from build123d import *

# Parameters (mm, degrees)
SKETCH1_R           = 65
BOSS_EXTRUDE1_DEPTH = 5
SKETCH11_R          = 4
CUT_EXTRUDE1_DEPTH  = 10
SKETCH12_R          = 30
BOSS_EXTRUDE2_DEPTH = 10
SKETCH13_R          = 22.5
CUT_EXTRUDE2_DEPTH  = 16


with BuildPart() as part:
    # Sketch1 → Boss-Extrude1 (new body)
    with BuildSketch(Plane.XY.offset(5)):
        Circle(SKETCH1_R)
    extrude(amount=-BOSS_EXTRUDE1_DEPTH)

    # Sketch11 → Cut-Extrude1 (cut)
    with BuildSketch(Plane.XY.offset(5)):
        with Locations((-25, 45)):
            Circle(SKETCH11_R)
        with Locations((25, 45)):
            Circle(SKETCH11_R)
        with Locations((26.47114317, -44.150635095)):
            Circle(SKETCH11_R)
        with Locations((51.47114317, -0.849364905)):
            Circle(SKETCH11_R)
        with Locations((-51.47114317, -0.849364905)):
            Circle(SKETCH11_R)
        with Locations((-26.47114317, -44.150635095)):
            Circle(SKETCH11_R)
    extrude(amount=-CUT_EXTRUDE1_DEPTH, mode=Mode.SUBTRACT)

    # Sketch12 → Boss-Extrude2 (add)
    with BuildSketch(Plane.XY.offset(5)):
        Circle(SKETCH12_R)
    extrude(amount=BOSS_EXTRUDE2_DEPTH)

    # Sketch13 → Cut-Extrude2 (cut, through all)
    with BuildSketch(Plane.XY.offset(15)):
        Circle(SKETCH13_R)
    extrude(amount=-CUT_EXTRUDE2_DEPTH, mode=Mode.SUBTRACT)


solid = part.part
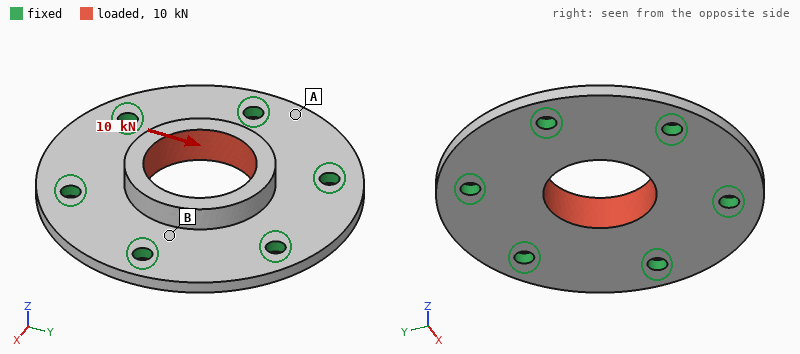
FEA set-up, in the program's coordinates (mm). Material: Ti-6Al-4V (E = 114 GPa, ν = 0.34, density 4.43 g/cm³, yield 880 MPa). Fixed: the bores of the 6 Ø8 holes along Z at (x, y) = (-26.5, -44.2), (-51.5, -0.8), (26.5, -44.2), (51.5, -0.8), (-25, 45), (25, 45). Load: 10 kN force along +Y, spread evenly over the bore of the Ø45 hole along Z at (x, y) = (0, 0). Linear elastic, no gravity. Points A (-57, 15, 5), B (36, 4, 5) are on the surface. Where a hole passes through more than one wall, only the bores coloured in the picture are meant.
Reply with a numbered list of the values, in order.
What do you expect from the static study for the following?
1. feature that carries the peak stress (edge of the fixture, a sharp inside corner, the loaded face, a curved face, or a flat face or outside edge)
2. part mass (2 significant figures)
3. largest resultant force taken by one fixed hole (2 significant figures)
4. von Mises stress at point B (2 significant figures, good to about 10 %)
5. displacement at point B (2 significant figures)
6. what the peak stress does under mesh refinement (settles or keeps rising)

1. edge of the fixture
2. 310 g
3. 2.1 kN
4. 12 MPa
5. 2.7 µm
6. keeps rising
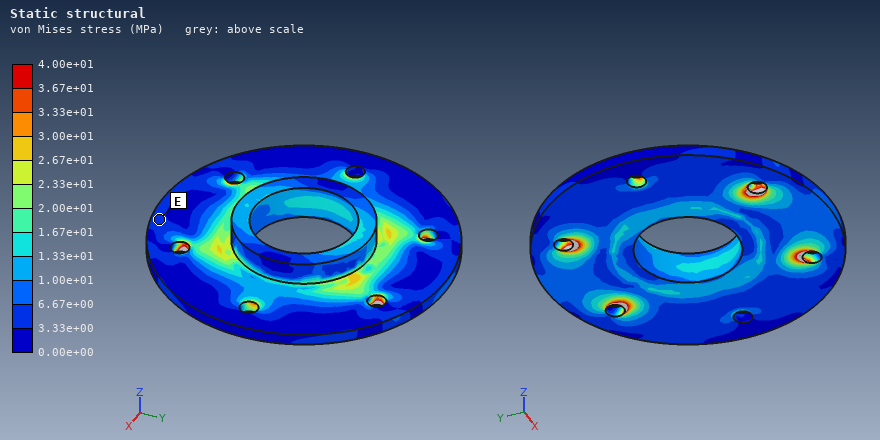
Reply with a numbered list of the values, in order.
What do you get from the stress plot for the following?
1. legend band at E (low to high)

1. 3.33e+00 to 6.67e+00 MPa
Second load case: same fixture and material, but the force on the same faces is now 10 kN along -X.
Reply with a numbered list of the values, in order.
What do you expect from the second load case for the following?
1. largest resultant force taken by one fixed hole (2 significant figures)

1. 2.3 kN
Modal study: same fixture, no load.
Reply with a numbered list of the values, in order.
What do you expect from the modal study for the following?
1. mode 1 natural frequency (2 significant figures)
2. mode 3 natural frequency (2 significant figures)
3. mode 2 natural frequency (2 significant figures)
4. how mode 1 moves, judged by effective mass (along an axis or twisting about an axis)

1. 6100 Hz
2. 7900 Hz
3. 7900 Hz
4. along Z
